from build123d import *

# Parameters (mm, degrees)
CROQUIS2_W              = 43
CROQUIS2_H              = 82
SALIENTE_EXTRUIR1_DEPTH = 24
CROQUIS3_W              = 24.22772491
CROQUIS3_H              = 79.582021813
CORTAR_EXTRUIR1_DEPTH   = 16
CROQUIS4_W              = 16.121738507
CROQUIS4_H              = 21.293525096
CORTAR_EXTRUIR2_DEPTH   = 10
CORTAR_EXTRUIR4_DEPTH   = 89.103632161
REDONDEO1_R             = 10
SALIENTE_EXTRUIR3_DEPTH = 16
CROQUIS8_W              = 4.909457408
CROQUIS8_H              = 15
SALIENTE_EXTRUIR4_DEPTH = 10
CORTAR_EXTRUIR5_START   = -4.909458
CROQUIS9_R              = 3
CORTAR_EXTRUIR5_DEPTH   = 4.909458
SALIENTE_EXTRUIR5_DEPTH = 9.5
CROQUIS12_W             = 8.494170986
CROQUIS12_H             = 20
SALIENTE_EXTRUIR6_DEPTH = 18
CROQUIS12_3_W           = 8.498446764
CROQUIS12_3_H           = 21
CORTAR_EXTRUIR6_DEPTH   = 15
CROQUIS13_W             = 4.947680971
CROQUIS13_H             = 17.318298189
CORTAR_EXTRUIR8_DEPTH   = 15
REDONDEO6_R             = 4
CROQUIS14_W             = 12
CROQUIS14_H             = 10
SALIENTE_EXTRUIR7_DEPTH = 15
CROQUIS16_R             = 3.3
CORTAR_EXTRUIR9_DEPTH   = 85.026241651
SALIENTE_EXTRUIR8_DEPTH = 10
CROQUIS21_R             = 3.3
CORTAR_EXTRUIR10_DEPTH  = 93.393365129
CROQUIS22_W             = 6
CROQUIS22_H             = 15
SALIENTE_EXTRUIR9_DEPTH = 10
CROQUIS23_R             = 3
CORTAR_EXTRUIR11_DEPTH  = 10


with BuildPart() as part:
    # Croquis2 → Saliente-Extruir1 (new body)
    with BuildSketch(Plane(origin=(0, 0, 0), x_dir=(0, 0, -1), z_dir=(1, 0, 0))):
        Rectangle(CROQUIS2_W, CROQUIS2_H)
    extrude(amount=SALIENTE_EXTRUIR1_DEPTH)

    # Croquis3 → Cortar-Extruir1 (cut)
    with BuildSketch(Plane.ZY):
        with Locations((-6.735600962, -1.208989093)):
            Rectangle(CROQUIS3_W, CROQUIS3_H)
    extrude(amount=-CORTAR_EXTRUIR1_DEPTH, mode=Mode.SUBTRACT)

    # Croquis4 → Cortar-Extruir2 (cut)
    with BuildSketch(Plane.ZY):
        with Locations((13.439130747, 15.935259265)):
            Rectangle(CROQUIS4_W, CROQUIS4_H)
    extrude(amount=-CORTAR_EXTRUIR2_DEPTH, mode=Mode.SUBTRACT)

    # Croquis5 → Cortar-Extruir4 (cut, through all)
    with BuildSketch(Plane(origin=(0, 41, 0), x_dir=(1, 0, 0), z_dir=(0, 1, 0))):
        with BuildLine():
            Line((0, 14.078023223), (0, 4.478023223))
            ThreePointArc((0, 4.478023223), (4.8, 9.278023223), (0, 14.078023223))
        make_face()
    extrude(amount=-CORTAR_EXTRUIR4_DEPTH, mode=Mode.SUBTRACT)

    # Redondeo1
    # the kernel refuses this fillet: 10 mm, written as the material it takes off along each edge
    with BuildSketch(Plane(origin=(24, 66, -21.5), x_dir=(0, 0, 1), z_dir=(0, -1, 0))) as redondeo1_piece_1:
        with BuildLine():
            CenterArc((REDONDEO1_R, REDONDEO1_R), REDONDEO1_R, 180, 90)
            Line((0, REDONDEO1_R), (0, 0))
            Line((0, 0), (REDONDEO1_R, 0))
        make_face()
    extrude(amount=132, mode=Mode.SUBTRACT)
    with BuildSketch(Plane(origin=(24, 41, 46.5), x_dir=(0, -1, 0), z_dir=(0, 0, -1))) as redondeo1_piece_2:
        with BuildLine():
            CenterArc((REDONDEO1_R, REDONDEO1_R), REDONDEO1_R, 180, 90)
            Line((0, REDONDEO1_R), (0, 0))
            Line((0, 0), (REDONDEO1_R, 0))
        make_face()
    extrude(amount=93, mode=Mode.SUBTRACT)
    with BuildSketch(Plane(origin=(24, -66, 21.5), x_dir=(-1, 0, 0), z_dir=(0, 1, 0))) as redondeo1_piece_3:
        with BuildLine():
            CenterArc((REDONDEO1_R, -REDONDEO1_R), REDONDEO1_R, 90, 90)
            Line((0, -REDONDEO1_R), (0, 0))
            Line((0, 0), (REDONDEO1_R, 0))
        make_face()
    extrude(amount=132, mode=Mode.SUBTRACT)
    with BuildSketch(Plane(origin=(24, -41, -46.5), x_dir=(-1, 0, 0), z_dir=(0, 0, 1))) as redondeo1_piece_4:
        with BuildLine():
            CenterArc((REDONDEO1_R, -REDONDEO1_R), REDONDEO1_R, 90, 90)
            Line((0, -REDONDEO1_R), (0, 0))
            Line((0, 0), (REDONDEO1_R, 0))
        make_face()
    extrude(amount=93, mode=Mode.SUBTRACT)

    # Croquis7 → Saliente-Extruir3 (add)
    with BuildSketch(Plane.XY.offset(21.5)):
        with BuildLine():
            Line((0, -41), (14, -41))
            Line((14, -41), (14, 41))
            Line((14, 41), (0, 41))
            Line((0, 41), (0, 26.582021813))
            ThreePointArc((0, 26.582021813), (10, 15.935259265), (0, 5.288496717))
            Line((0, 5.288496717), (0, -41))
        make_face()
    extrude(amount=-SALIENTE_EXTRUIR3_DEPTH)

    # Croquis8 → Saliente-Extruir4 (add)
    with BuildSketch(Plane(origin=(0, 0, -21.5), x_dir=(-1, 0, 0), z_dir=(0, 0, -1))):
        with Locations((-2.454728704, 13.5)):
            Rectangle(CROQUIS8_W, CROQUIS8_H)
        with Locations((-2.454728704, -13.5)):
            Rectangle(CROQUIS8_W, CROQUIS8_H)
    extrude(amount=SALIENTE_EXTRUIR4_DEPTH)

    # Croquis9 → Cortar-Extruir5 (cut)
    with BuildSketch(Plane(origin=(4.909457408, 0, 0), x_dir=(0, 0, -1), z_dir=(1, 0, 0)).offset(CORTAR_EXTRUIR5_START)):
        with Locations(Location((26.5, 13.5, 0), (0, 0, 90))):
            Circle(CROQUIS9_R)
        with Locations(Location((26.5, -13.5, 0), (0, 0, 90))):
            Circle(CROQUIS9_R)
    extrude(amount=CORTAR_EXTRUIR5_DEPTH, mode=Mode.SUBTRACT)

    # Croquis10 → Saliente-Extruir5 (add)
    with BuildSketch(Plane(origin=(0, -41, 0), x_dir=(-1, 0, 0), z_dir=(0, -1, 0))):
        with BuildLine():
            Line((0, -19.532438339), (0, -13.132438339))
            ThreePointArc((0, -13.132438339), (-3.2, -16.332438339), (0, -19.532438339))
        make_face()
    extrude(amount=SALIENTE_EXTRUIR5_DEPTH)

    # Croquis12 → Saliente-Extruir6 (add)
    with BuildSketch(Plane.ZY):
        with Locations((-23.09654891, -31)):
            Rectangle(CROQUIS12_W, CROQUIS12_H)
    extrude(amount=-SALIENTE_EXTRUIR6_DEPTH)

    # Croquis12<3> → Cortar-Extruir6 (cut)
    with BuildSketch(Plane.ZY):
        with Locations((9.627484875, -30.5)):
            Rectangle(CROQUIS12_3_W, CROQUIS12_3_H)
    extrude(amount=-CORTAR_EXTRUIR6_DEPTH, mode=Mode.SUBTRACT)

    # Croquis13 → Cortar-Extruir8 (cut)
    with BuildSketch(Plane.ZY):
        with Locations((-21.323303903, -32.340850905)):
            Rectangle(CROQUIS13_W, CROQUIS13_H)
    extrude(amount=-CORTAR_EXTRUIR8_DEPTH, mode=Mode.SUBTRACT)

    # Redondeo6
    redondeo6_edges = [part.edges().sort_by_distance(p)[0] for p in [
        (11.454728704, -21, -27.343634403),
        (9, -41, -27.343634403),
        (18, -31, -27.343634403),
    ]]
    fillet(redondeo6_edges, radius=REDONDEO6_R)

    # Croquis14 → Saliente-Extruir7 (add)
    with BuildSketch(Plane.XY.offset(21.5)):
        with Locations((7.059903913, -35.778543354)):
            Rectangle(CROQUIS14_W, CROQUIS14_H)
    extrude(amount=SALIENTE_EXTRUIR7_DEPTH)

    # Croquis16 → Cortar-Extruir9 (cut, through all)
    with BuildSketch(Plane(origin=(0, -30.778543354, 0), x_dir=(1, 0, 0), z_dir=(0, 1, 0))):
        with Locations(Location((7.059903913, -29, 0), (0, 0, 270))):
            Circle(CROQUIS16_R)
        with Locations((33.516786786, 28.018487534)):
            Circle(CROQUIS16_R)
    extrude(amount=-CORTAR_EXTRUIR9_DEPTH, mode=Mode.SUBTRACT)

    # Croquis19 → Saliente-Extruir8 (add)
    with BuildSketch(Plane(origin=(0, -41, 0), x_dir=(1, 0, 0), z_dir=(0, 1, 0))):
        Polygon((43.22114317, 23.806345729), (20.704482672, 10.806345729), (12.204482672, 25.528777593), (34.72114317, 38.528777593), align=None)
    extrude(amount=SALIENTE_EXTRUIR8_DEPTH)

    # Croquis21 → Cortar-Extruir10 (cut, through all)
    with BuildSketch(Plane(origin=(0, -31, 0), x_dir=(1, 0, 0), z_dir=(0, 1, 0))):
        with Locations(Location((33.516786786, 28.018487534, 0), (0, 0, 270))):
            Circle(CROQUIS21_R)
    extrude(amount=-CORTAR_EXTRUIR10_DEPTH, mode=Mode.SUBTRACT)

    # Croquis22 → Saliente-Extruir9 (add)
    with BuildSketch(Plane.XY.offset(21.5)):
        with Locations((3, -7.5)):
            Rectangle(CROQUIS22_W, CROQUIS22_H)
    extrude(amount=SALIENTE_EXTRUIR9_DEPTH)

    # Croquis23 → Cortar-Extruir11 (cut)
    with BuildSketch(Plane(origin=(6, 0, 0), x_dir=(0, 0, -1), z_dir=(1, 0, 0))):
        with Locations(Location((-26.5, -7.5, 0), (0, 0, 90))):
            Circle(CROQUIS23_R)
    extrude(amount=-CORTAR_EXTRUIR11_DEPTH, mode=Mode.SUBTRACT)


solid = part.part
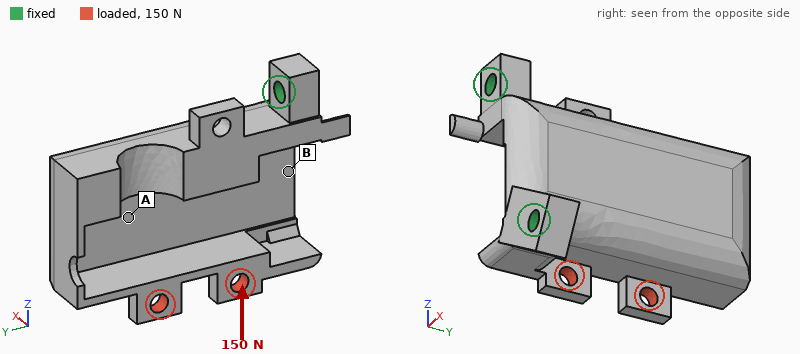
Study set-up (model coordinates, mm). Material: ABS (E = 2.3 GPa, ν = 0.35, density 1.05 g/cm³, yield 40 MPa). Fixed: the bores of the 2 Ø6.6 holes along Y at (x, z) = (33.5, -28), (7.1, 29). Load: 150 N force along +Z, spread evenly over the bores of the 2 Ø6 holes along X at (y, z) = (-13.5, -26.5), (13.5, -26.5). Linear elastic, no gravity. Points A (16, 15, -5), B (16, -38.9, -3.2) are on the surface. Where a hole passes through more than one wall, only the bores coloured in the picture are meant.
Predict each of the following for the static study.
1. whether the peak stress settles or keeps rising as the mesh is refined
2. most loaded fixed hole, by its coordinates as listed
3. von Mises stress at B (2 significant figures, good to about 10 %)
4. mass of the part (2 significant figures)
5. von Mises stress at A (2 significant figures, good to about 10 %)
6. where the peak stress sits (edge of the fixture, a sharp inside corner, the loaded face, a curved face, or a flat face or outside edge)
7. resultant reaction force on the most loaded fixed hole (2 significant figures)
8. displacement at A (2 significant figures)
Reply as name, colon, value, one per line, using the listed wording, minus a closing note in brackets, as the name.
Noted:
whether the peak stress settles or keeps rising as the mesh is refined: keeps rising
most loaded fixed hole, by its coordinates as listed: (7.1, 29)
von Mises stress at B: 1.3 MPa
mass of the part: 54 g
von Mises stress at A: 2.3 MPa
where the peak stress sits: a sharp inside corner
resultant reaction force on the most loaded fixed hole: 140 N
displacement at A: 0.26 mm
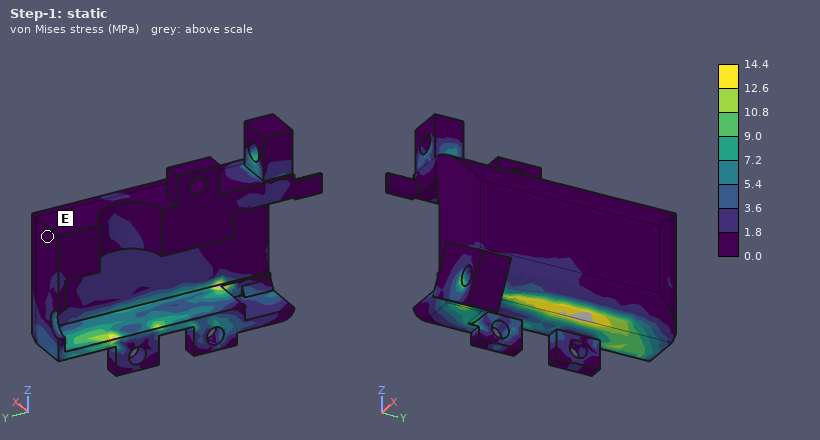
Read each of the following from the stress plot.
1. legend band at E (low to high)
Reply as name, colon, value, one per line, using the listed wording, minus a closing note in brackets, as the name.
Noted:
legend band at E: 0.0 to 1.8 MPa
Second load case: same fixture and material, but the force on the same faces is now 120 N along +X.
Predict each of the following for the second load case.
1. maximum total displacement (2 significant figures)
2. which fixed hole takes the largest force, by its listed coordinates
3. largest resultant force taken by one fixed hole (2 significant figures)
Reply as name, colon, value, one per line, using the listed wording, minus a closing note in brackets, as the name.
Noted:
maximum total displacement: 1.5 mm
which fixed hole takes the largest force, by its listed coordinates: (33.5, -28)
largest resultant force taken by one fixed hole: 130 N
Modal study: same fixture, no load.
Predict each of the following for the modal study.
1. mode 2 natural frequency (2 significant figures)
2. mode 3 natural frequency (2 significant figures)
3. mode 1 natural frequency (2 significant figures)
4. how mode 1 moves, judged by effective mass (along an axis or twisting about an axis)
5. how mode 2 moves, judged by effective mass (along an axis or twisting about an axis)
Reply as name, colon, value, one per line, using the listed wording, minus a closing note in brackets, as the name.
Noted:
mode 2 natural frequency: 810 Hz
mode 3 natural frequency: 1000 Hz
mode 1 natural frequency: 290 Hz
how mode 1 moves, judged by effective mass: along X
how mode 2 moves, judged by effective mass: along Z
